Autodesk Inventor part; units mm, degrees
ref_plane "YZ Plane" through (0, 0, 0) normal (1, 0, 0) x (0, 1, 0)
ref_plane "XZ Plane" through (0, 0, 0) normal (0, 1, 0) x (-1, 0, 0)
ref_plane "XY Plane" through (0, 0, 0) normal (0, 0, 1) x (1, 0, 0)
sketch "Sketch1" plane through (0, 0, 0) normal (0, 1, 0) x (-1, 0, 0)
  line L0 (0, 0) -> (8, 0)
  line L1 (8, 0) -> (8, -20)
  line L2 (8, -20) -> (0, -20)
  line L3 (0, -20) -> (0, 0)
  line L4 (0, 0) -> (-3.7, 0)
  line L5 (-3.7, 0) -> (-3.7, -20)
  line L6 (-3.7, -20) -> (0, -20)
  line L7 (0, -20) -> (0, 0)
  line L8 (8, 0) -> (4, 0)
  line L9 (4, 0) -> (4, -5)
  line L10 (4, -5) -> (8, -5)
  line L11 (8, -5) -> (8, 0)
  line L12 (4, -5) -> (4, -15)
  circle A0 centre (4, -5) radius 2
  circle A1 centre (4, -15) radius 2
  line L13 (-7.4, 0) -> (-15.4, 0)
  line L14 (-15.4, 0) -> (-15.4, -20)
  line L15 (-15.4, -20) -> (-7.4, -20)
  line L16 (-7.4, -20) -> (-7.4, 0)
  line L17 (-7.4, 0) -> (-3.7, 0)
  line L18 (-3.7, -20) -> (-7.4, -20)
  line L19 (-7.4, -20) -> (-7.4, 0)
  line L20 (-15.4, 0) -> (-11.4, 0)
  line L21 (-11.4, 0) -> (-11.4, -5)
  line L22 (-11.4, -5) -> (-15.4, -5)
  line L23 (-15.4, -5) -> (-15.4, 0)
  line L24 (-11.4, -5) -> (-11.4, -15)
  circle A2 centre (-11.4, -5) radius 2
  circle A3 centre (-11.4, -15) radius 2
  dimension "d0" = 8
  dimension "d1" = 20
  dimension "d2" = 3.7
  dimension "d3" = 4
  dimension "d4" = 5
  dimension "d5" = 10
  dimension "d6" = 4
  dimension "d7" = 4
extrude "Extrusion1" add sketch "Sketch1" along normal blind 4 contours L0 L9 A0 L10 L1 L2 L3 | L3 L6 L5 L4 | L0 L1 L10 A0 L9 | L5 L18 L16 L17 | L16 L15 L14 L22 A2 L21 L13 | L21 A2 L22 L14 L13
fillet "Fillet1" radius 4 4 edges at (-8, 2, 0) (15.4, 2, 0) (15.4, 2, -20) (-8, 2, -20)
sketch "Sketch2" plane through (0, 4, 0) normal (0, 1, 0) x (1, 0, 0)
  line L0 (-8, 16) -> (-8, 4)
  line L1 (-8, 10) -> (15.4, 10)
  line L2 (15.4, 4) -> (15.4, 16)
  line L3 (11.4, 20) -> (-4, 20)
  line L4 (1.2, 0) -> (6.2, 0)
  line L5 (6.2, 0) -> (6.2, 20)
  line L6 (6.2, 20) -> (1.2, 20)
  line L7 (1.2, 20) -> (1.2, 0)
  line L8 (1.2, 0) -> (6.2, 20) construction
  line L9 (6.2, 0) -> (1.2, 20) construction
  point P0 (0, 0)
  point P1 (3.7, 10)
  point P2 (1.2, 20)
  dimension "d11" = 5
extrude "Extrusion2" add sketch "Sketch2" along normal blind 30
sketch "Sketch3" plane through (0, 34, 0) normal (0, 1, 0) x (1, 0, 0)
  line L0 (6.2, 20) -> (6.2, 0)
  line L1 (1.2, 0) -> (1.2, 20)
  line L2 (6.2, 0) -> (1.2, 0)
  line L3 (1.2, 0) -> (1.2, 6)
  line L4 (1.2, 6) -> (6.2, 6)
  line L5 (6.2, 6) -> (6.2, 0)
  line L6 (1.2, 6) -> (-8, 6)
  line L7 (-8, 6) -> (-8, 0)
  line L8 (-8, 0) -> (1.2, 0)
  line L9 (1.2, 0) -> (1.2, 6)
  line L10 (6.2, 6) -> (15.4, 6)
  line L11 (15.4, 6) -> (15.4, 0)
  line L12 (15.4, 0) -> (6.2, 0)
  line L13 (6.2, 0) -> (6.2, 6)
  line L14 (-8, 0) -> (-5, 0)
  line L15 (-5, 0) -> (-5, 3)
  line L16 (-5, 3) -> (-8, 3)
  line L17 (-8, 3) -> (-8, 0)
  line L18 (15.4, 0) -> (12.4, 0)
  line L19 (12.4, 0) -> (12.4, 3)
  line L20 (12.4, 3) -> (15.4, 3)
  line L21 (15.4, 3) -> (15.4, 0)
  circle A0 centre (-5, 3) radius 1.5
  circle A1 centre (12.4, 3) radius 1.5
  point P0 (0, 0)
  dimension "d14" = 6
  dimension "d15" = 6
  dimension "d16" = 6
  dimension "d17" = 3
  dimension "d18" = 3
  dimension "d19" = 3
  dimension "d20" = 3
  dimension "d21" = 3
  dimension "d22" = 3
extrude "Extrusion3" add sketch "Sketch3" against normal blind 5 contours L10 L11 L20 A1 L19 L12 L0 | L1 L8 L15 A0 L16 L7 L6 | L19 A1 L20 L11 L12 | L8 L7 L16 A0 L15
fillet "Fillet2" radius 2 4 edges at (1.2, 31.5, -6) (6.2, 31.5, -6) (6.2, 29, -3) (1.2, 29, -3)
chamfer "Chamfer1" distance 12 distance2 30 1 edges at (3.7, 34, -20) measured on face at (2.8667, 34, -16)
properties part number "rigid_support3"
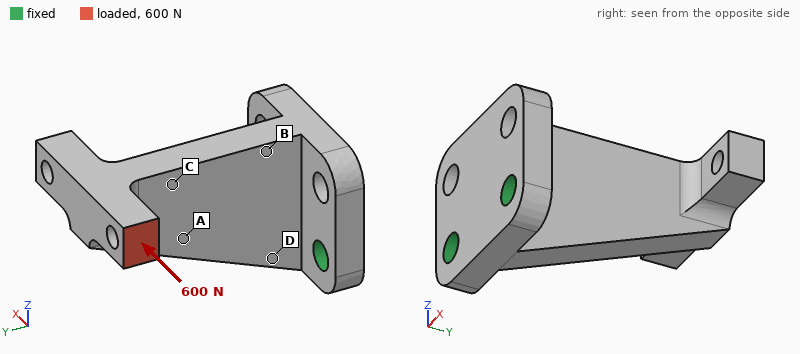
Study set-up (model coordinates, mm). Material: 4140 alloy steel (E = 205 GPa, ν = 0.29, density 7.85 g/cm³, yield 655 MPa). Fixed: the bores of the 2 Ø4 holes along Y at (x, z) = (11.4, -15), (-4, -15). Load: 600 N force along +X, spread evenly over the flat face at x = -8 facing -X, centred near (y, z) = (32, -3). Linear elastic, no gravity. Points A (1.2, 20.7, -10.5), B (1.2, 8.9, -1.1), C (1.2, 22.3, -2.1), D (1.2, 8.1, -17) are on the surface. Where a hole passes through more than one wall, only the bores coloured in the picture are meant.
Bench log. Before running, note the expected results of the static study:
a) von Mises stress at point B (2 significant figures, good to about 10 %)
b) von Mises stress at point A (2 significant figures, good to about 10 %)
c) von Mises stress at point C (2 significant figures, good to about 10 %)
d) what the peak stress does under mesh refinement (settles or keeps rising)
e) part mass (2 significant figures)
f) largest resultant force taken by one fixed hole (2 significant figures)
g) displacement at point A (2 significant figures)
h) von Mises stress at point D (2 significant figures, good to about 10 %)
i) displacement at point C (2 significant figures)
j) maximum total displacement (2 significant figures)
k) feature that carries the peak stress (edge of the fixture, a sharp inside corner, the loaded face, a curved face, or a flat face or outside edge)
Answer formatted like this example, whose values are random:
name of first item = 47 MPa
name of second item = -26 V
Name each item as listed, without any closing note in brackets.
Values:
von Mises stress at point B = 180 MPa
von Mises stress at point A = 130 MPa
von Mises stress at point C = 110 MPa
what the peak stress does under mesh refinement = keeps rising
part mass = 33 g
largest resultant force taken by one fixed hole = 1.5 kN
displacement at point A = 0.078 mm
von Mises stress at point D = 200 MPa
displacement at point C = 0.10 mm
maximum total displacement = 0.23 mm
feature that carries the peak stress = edge of the fixture
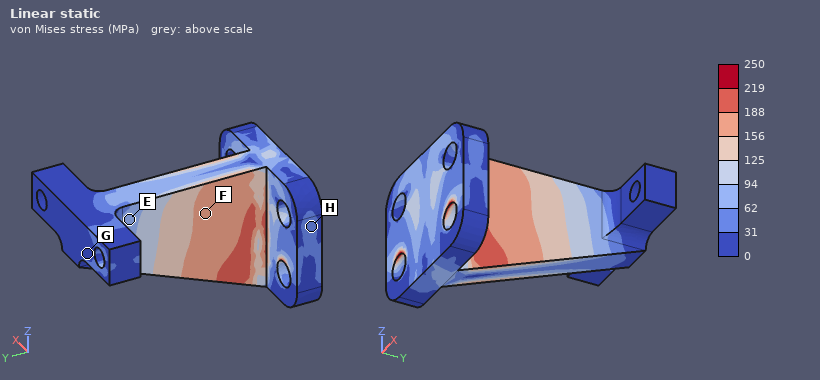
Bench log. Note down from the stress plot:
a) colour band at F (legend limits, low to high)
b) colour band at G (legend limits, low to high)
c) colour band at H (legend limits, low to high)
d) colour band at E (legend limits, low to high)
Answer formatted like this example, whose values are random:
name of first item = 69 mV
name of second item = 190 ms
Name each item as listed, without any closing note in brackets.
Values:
colour band at F = 156 to 188 MPa
colour band at G = 0 to 31 MPa
colour band at H = 31 to 62 MPa
colour band at E = 62 to 94 MPa
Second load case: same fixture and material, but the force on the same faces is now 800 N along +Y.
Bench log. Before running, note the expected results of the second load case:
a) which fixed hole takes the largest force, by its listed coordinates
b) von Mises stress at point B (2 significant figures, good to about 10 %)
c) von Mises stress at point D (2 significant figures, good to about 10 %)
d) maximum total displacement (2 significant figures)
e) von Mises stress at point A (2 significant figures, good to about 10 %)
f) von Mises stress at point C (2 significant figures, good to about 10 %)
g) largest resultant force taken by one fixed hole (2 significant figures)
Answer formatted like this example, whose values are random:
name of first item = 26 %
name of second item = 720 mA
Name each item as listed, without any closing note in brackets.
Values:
which fixed hole takes the largest force, by its listed coordinates = (-4, -15)
von Mises stress at point B = 140 MPa
von Mises stress at point D = 100 MPa
maximum total displacement = 0.23 mm
von Mises stress at point A = 170 MPa
von Mises stress at point C = 210 MPa
largest resultant force taken by one fixed hole = 1.2 kN
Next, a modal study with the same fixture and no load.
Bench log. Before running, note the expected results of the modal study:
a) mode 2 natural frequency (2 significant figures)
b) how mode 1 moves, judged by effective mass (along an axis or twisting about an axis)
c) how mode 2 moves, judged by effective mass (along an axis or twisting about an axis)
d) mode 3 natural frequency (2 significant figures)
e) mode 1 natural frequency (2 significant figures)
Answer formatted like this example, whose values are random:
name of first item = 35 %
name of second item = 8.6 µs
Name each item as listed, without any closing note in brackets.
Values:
mode 2 natural frequency = 4300 Hz
how mode 1 moves, judged by effective mass = along X
how mode 2 moves, judged by effective mass = along Z
mode 3 natural frequency = 11 kHz
mode 1 natural frequency = 3200 Hz
